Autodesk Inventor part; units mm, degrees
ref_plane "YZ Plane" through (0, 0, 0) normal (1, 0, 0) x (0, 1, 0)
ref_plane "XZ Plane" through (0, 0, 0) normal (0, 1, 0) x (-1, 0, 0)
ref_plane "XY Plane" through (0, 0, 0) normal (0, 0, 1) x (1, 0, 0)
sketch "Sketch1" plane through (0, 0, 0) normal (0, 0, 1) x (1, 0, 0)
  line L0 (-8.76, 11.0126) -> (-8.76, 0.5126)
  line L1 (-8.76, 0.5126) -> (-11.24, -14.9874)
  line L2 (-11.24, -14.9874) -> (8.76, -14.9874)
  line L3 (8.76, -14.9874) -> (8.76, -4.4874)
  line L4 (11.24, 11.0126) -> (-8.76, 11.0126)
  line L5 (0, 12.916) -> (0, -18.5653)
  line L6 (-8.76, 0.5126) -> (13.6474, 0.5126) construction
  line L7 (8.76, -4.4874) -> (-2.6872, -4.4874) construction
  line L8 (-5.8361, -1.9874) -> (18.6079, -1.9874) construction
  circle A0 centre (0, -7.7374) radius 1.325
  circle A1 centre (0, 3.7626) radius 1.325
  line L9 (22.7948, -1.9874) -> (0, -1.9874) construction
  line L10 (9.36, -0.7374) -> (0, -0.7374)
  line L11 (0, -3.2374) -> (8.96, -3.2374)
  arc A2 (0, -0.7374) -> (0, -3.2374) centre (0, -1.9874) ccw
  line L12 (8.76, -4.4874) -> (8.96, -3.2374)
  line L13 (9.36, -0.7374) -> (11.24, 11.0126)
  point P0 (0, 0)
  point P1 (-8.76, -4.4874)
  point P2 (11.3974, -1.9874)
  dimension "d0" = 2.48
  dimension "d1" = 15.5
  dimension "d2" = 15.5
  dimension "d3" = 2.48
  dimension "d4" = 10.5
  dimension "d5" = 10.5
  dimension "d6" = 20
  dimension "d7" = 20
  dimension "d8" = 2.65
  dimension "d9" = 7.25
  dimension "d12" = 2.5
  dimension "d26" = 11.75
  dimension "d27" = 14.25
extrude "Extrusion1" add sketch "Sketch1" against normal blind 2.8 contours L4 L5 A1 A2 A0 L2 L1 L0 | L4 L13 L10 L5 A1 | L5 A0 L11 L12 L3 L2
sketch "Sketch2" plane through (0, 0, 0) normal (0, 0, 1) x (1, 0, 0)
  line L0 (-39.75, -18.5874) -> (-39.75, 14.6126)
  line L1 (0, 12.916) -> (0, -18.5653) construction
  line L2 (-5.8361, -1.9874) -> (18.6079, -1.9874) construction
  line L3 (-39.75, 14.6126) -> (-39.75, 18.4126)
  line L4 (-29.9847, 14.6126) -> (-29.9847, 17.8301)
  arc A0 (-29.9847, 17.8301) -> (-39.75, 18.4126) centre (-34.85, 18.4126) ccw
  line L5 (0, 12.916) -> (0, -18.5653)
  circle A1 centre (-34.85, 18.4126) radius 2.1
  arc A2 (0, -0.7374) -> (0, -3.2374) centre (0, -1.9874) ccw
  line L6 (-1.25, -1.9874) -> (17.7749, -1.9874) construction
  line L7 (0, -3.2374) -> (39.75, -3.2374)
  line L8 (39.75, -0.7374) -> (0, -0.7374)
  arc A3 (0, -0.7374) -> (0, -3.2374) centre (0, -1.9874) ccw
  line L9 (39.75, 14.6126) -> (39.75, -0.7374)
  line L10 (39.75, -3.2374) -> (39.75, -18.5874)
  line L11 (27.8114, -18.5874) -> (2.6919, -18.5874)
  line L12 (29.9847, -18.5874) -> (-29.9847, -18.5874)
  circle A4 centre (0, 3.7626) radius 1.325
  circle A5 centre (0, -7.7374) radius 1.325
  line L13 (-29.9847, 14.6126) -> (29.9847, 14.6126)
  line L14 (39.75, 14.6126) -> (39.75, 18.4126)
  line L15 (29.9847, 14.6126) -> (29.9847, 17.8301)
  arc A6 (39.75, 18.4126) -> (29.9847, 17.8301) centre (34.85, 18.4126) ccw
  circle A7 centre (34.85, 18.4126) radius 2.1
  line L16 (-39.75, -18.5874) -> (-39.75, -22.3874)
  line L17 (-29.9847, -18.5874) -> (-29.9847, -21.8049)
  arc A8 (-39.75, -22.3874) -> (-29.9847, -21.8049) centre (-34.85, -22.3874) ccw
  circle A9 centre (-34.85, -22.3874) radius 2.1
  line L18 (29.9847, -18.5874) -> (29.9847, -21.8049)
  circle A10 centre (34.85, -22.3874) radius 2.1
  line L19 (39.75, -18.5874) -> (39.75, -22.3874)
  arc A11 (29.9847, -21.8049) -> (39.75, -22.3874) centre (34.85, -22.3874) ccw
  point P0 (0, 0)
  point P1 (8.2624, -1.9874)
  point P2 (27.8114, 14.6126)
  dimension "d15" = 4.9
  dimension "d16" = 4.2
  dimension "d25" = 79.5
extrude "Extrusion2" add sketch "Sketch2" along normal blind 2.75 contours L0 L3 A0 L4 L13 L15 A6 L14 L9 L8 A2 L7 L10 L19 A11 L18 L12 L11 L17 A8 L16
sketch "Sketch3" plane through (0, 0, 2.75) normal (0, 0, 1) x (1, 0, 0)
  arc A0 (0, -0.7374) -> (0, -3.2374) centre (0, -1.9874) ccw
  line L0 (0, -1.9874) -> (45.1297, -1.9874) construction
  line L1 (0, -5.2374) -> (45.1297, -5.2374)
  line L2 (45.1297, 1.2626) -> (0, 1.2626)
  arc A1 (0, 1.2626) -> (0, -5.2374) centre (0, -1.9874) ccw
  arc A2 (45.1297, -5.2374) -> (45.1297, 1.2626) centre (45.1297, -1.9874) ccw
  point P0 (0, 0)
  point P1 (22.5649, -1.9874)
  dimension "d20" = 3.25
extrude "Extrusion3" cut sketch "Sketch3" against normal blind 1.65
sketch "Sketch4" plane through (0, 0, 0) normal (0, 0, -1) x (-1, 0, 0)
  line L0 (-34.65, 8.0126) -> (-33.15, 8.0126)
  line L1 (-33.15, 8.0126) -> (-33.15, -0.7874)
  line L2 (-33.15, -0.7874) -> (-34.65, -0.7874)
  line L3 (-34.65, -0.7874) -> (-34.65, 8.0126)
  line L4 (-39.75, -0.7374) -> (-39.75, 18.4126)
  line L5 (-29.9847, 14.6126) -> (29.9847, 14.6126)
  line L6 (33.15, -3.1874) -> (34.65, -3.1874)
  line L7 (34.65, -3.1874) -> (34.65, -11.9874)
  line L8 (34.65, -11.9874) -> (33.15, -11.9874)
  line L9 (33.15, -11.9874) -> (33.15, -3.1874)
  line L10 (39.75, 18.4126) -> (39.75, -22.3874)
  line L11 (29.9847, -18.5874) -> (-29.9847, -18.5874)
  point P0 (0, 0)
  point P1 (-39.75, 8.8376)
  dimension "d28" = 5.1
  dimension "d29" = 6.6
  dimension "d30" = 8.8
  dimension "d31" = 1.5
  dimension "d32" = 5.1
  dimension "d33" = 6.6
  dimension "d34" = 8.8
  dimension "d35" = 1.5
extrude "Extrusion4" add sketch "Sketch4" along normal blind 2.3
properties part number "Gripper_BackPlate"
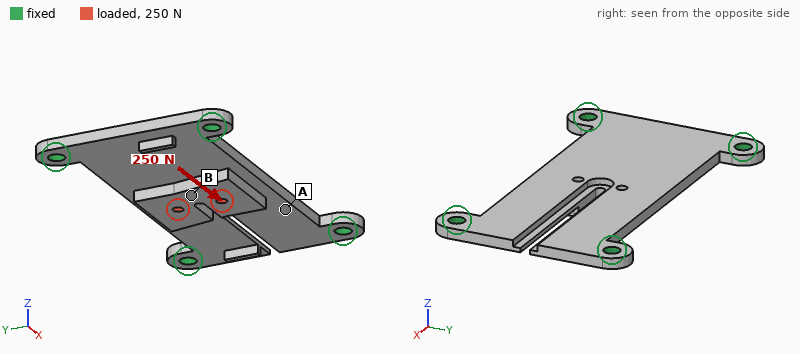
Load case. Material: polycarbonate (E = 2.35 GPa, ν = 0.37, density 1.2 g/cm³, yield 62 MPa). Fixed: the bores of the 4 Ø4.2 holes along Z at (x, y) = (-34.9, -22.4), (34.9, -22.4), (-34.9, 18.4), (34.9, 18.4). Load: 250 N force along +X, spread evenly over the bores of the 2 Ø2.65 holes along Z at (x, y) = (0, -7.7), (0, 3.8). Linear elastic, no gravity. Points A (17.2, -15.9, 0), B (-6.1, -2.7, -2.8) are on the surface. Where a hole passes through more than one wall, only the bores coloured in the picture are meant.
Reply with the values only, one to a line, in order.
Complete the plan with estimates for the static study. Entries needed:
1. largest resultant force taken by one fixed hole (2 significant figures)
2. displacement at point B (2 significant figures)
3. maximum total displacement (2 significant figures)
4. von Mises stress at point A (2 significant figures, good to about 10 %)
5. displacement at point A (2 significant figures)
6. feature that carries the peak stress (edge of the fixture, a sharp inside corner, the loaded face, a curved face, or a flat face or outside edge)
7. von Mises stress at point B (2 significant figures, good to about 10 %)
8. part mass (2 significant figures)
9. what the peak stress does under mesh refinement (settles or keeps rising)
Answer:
75 N
0.094 mm
0.18 mm
5.1 MPa
0.13 mm
edge of the fixture
0.93 MPa
10 g
keeps rising
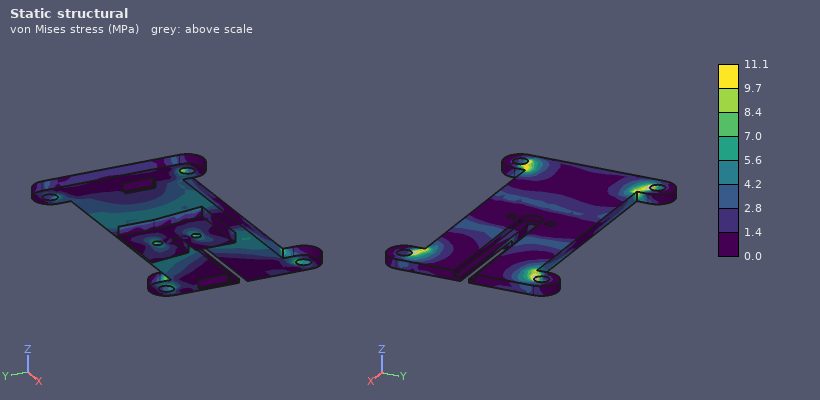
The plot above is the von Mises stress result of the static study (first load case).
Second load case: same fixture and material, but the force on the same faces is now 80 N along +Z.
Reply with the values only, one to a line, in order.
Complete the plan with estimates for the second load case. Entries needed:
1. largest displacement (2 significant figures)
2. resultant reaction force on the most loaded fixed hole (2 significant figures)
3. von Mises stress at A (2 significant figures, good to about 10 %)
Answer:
0.95 mm
30 N
6.8 MPa
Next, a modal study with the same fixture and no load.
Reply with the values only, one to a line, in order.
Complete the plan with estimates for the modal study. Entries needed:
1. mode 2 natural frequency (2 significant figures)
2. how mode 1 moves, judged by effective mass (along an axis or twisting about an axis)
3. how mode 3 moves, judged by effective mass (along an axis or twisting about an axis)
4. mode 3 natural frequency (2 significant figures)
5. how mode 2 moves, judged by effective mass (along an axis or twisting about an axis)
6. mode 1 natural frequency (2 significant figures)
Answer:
1200 Hz
along Z
twisting about Y
1600 Hz
twisting about X
660 Hz
